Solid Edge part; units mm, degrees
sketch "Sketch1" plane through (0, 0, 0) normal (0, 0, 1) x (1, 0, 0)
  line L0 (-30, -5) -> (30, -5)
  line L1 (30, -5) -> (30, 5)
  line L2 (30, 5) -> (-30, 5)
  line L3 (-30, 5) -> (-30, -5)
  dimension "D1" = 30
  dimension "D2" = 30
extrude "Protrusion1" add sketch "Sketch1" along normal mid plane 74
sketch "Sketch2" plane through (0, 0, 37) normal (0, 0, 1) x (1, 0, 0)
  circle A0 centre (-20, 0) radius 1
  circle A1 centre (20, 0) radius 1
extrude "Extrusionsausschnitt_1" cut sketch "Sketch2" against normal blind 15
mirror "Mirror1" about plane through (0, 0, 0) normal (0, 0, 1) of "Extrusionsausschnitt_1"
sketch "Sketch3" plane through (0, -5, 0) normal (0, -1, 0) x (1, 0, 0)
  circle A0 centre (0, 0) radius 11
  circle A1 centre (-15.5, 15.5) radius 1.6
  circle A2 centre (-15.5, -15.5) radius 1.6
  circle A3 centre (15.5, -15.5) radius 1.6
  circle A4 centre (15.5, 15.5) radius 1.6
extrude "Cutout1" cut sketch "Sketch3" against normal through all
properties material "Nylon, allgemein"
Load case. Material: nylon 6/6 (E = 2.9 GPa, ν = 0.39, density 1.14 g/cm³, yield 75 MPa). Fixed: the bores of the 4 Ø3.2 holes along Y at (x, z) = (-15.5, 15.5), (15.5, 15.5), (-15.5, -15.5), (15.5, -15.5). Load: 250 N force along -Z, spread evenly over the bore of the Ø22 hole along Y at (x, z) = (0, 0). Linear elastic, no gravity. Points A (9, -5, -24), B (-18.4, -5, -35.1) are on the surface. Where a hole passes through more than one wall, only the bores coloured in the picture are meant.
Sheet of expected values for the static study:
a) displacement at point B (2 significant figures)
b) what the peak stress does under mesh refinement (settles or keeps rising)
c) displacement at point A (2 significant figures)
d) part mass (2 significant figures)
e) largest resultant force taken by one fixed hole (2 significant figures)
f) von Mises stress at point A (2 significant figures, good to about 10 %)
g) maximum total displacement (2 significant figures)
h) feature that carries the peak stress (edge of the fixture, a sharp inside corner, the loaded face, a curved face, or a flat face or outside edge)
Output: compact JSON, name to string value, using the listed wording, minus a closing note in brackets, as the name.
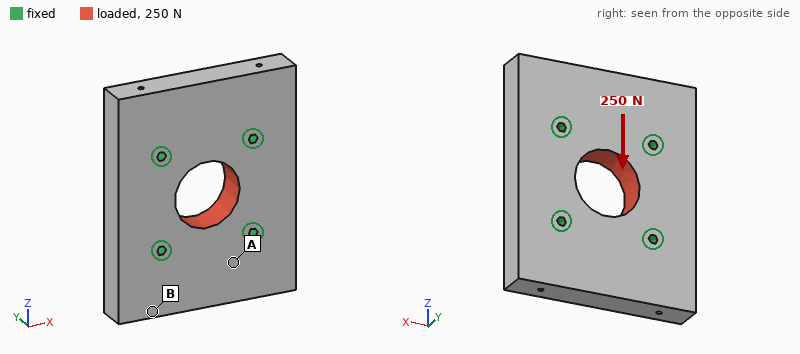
{"displacement at point B": "0.84 µm", "what the peak stress does under mesh refinement": "keeps rising", "displacement at point A": "1.4 µm", "part mass": "46 g", "largest resultant force taken by one fixed hole": "63 N", "von Mises stress at point A": "0.24 MPa", "maximum total displacement": "3.2 µm", "feature that carries the peak stress": "edge of the fixture"}
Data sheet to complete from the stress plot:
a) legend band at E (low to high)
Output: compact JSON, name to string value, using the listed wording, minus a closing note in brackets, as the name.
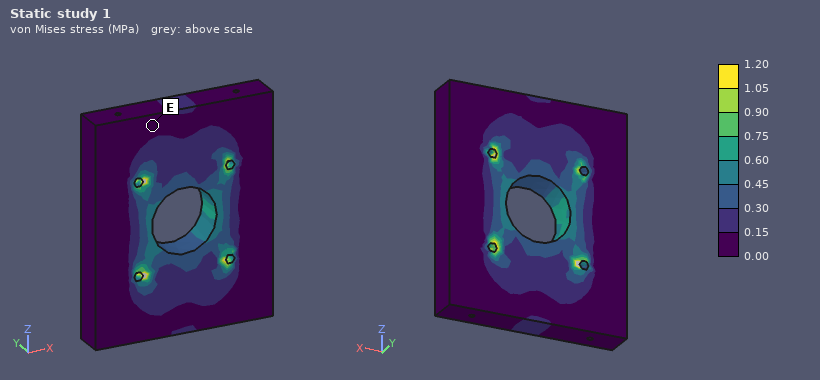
{"legend band at E": "0.00 to 0.15 MPa"}
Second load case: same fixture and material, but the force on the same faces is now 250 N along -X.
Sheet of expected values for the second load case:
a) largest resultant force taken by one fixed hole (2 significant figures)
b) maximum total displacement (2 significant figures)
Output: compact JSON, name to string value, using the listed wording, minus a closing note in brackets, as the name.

{"largest resultant force taken by one fixed hole": "64 N", "maximum total displacement": "3.6 µm"}
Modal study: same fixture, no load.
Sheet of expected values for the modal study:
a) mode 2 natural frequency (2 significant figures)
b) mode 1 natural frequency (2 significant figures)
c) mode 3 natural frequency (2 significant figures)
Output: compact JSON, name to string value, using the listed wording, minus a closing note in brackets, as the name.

{"mode 2 natural frequency": "3800 Hz", "mode 1 natural frequency": "3700 Hz", "mode 3 natural frequency": "4700 Hz"}
